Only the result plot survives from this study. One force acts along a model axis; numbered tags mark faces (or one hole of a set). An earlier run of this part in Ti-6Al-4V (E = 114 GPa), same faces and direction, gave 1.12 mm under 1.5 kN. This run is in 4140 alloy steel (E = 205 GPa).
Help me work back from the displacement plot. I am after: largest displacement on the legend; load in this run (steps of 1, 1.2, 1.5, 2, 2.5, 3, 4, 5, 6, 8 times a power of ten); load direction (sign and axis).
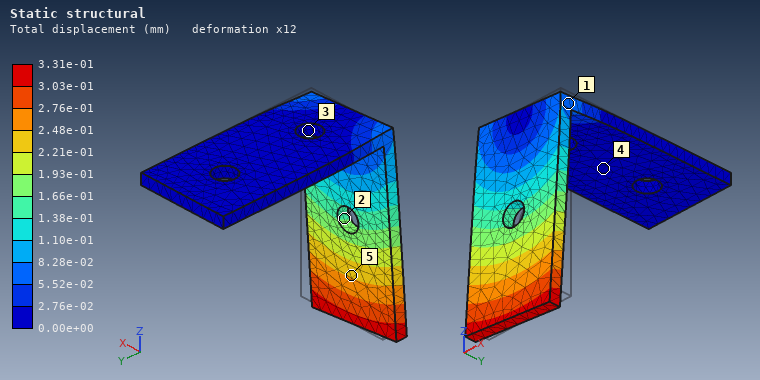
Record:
3.31e-01 mm
800 N
-X
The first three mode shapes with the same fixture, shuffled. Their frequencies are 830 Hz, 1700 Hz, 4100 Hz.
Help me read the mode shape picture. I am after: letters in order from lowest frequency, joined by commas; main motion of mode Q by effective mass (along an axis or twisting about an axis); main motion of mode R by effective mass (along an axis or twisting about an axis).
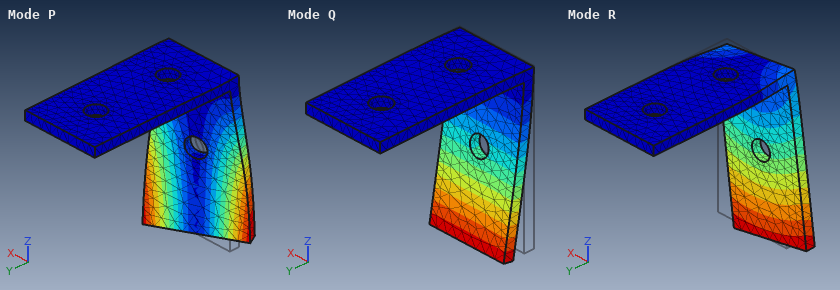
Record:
Q, R, P
along Y
along X
